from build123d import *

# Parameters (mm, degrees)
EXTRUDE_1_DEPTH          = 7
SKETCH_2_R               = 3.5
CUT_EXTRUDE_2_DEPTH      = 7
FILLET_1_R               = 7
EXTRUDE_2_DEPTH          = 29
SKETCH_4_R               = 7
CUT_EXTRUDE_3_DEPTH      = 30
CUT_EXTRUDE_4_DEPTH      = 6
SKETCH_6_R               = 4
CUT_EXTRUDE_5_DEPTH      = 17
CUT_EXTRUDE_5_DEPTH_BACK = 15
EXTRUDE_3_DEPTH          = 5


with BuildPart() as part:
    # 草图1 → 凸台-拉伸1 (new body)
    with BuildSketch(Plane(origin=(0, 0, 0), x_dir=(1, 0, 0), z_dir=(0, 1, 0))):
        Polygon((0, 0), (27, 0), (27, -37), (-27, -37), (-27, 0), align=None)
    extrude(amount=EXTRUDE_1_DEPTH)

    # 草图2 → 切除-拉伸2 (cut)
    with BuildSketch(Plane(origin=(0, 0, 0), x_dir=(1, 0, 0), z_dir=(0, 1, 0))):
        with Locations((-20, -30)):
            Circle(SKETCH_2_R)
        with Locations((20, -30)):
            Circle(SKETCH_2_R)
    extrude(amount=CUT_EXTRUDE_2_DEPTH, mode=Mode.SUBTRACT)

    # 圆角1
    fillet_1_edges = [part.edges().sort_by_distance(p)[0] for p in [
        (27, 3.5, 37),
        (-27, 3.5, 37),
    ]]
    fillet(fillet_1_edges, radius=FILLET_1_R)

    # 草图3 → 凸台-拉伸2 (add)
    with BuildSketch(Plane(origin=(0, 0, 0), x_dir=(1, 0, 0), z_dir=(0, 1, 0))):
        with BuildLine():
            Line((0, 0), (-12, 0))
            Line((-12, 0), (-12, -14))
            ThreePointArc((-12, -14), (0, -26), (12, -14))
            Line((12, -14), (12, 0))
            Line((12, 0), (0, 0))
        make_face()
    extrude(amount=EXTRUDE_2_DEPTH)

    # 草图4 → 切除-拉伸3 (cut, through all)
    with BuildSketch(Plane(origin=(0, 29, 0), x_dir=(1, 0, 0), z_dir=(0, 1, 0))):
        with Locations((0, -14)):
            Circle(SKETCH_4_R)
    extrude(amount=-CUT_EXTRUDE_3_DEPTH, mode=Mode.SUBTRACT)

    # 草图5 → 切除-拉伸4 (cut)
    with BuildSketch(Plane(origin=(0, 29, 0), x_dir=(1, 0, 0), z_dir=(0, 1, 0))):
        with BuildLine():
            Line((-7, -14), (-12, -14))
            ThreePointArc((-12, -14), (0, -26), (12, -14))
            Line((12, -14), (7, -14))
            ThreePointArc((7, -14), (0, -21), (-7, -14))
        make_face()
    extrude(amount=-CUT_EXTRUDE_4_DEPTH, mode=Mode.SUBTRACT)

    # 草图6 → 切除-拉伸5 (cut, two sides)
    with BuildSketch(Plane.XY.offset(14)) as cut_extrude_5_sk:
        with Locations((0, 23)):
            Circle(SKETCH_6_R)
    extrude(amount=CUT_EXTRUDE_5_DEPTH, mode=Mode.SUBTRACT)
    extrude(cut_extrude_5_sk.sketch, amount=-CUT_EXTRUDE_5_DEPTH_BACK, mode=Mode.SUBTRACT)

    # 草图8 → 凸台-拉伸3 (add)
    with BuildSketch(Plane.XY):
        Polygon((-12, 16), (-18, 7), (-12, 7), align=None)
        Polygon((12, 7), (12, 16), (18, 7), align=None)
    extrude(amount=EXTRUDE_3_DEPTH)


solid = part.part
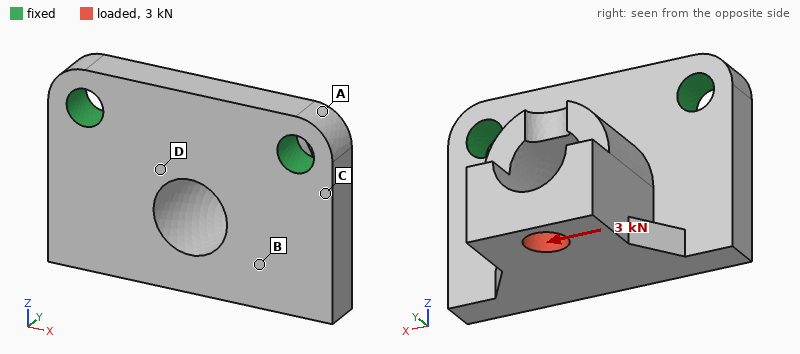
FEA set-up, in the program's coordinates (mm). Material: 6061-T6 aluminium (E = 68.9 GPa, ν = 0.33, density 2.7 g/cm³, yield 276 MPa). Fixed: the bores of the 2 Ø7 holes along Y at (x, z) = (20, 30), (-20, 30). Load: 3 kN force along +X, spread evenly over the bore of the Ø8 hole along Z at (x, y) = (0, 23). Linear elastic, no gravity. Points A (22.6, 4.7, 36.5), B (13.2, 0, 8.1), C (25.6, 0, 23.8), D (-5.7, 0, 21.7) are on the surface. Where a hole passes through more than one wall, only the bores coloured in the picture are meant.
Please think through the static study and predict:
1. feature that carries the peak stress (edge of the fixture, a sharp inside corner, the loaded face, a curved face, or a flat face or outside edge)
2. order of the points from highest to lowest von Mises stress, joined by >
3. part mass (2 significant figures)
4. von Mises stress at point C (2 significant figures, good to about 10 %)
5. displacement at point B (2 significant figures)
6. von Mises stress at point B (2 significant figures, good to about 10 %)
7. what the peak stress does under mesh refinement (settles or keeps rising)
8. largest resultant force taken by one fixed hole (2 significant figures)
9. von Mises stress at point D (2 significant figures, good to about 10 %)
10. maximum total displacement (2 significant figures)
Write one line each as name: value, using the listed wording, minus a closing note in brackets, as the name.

feature that carries the peak stress: edge of the fixture
order of the points from highest to lowest von Mises stress, joined by >: C > B > D > A
part mass: 54 g
von Mises stress at point C: 56 MPa
displacement at point B: 27 µm
von Mises stress at point B: 36 MPa
what the peak stress does under mesh refinement: keeps rising
largest resultant force taken by one fixed hole: 2.9 kN
von Mises stress at point D: 25 MPa
maximum total displacement: 89 µm
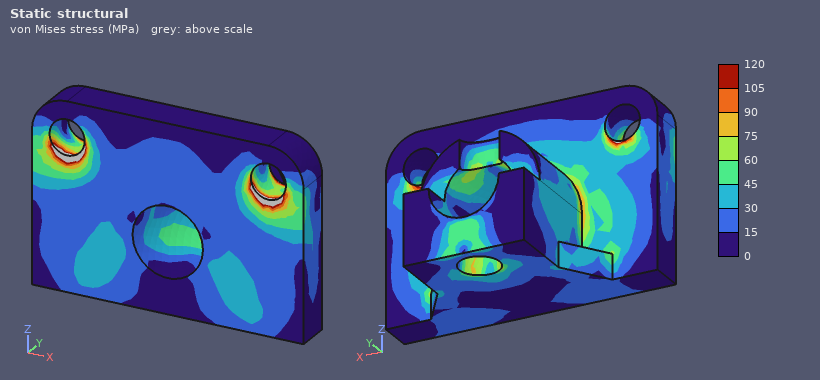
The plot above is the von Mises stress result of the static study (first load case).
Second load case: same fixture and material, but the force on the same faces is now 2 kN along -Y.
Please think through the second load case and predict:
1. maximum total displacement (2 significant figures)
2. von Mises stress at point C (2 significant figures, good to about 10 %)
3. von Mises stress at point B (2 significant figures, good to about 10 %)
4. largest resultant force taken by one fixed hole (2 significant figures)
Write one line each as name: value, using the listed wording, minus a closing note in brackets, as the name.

maximum total displacement: 0.20 mm
von Mises stress at point C: 93 MPa
von Mises stress at point B: 24 MPa
largest resultant force taken by one fixed hole: 1.0 kN
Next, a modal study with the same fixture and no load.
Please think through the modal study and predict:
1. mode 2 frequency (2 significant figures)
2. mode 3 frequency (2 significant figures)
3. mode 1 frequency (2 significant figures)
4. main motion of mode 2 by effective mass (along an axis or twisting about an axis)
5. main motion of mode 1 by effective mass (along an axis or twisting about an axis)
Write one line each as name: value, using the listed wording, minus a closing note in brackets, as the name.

mode 2 frequency: 8400 Hz
mode 3 frequency: 14 kHz
mode 1 frequency: 3600 Hz
main motion of mode 2 by effective mass: along X
main motion of mode 1 by effective mass: along Y
